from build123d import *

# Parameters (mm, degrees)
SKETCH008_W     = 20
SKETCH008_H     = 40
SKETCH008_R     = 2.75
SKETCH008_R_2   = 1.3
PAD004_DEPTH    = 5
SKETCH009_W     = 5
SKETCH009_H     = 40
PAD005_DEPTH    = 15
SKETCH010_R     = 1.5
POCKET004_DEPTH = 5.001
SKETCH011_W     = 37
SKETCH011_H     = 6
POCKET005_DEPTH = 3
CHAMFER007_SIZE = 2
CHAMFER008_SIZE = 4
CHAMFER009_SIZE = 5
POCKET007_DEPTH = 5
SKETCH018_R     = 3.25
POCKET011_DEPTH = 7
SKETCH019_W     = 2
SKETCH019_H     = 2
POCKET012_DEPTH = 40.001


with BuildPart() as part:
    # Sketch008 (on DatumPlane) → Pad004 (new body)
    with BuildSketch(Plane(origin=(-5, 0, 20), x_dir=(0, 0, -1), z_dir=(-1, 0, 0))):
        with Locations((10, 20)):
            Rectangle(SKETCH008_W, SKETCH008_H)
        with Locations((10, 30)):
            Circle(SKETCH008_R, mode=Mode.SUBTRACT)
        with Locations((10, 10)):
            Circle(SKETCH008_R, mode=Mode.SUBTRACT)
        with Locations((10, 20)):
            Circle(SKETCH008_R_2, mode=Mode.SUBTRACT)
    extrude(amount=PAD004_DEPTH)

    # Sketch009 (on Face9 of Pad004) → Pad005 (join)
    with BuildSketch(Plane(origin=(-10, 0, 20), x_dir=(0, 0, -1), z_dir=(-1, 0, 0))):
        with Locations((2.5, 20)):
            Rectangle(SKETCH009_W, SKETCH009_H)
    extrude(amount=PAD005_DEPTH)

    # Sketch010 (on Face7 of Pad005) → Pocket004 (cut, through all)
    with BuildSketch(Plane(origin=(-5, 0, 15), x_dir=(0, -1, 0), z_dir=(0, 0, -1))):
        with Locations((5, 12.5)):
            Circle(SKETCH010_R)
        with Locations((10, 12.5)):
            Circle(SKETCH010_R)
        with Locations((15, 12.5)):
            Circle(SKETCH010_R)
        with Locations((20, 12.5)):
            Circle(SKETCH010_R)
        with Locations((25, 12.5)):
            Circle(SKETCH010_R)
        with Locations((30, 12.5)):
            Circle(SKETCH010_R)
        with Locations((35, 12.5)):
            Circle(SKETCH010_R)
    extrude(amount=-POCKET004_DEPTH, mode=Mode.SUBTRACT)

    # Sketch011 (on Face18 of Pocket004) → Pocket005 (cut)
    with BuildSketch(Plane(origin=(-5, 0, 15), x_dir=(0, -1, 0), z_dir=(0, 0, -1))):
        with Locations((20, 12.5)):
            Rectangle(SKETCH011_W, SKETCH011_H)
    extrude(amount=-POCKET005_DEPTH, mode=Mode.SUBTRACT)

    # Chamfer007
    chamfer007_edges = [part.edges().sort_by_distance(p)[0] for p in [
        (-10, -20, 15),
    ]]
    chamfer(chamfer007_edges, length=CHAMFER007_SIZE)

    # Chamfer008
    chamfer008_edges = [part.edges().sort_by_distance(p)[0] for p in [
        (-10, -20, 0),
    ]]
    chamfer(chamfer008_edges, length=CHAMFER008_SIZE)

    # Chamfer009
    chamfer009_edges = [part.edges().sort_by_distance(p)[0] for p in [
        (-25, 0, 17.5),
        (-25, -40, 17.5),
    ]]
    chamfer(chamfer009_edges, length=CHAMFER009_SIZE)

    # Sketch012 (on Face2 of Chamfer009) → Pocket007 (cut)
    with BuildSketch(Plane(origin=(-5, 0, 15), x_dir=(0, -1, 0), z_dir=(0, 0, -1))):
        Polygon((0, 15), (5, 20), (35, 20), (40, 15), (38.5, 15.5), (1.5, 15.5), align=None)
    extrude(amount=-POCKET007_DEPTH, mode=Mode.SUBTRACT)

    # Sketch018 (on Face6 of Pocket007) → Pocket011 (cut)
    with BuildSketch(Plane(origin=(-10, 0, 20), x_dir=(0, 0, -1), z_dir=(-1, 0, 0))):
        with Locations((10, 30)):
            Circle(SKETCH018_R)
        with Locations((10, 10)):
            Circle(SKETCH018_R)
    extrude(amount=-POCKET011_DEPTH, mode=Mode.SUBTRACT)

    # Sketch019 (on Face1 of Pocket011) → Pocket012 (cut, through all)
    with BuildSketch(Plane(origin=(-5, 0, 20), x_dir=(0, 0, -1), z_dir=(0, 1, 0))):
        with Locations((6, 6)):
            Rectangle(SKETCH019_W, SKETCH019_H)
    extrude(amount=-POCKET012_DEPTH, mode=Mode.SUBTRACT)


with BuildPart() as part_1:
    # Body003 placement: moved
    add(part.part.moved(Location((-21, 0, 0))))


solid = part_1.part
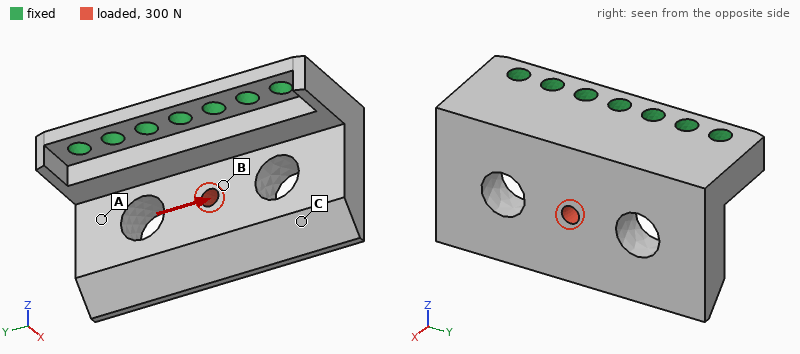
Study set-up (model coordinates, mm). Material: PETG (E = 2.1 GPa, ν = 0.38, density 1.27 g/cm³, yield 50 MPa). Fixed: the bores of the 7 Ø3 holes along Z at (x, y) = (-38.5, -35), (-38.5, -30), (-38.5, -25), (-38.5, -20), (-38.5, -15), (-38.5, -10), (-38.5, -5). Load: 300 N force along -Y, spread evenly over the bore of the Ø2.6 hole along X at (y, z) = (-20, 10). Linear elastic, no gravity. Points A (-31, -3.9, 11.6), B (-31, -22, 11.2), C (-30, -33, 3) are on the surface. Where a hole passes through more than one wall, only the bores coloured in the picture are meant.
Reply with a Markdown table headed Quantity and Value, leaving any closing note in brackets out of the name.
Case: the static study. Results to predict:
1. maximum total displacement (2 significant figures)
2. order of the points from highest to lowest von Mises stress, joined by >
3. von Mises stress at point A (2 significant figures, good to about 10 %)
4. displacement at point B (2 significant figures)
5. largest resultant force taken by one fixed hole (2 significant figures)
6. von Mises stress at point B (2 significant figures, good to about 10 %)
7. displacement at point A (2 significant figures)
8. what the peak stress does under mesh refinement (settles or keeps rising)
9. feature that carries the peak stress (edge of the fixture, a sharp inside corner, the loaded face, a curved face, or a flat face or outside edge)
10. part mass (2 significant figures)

| Quantity | Value |
|---|---|
| maximum total displacement | 0.31 mm |
| order of the points from highest to lowest von Mises stress, joined by > | B > A > C |
| von Mises stress at point A | 5.5 MPa |
| displacement at point B | 0.12 mm |
| largest resultant force taken by one fixed hole | 100 N |
| von Mises stress at point B | 9.5 MPa |
| displacement at point A | 0.16 mm |
| what the peak stress does under mesh refinement | keeps rising |
| feature that carries the peak stress | edge of the fixture |
| part mass | 5.9 g |
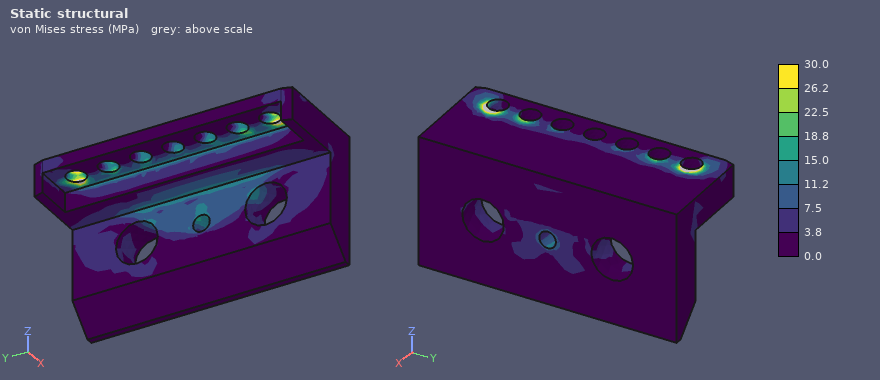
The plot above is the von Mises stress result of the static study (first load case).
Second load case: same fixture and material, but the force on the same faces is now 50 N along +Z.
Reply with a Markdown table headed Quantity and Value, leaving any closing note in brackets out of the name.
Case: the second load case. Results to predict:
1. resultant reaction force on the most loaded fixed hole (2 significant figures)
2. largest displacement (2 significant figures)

| Quantity | Value |
|---|---|
| resultant reaction force on the most loaded fixed hole | 8.2 N |
| largest displacement | 0.35 mm |
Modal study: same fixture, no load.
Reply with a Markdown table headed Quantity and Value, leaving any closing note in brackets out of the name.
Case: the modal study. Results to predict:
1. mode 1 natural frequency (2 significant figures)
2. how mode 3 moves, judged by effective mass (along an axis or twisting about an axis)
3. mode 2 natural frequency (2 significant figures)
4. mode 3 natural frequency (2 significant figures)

| Quantity | Value |
|---|---|
| mode 1 natural frequency | 930 Hz |
| how mode 3 moves, judged by effective mass | along Y |
| mode 2 natural frequency | 2100 Hz |
| mode 3 natural frequency | 4300 Hz |
